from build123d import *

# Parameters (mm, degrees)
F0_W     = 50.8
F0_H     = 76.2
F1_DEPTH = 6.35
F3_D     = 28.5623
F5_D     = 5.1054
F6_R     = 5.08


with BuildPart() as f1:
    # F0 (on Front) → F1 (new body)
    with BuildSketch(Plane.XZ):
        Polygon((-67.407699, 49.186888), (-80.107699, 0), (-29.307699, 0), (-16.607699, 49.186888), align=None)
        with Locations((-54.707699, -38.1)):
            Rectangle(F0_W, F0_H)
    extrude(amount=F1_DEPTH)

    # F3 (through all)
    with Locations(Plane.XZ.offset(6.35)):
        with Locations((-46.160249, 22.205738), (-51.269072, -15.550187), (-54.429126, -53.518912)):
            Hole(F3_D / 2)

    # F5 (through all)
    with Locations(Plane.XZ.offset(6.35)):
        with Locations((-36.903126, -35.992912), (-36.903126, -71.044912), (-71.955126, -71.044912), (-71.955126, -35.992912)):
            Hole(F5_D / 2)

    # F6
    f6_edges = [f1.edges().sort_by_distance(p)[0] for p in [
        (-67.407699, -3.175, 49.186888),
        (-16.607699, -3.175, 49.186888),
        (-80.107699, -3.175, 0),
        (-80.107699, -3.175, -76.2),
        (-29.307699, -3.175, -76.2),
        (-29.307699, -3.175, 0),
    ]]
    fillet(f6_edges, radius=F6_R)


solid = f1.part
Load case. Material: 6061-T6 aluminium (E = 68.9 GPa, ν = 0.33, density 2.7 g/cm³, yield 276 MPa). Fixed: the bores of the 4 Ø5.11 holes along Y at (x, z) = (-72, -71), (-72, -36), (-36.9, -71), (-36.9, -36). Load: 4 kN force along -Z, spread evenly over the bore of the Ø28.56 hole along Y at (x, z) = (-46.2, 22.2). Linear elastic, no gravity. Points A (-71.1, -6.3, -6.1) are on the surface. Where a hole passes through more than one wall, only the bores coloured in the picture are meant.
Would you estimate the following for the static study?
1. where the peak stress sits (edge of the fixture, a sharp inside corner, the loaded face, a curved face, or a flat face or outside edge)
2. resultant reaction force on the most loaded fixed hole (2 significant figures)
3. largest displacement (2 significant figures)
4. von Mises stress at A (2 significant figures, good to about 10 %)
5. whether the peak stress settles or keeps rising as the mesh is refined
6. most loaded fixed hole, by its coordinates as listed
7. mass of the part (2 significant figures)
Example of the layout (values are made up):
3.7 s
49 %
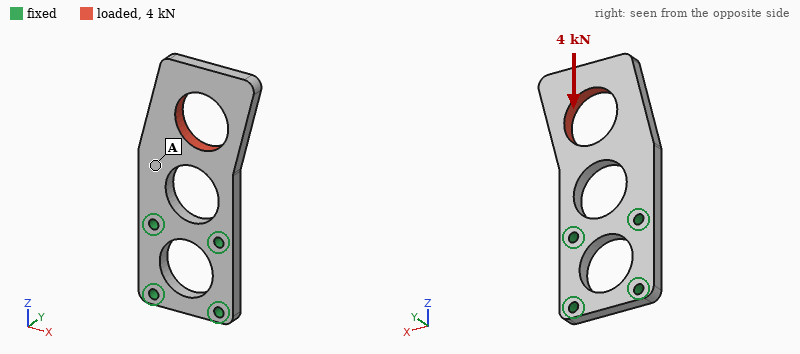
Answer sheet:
edge of the fixture
2.6 kN
73 µm
15 MPa
keeps rising
(-36.9, -36)
74 g
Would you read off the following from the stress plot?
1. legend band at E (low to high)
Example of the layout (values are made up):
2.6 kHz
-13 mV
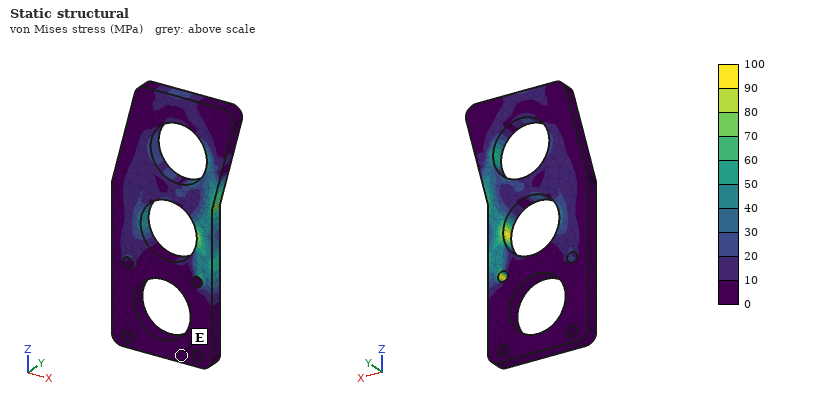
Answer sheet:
0 to 10 MPa
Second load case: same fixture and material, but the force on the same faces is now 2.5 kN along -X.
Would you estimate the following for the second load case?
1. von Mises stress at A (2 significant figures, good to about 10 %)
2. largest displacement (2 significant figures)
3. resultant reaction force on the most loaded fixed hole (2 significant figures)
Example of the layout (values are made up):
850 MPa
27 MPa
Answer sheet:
26 MPa
0.21 mm
3.3 kN
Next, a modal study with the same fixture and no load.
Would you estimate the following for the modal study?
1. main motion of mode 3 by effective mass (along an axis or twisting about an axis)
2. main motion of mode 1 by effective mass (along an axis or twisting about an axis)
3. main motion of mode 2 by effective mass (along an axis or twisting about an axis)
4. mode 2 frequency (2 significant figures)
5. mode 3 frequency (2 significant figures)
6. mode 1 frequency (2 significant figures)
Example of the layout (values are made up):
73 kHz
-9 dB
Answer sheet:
along X
along Y
twisting about Z
2000 Hz
3200 Hz
600 Hz
